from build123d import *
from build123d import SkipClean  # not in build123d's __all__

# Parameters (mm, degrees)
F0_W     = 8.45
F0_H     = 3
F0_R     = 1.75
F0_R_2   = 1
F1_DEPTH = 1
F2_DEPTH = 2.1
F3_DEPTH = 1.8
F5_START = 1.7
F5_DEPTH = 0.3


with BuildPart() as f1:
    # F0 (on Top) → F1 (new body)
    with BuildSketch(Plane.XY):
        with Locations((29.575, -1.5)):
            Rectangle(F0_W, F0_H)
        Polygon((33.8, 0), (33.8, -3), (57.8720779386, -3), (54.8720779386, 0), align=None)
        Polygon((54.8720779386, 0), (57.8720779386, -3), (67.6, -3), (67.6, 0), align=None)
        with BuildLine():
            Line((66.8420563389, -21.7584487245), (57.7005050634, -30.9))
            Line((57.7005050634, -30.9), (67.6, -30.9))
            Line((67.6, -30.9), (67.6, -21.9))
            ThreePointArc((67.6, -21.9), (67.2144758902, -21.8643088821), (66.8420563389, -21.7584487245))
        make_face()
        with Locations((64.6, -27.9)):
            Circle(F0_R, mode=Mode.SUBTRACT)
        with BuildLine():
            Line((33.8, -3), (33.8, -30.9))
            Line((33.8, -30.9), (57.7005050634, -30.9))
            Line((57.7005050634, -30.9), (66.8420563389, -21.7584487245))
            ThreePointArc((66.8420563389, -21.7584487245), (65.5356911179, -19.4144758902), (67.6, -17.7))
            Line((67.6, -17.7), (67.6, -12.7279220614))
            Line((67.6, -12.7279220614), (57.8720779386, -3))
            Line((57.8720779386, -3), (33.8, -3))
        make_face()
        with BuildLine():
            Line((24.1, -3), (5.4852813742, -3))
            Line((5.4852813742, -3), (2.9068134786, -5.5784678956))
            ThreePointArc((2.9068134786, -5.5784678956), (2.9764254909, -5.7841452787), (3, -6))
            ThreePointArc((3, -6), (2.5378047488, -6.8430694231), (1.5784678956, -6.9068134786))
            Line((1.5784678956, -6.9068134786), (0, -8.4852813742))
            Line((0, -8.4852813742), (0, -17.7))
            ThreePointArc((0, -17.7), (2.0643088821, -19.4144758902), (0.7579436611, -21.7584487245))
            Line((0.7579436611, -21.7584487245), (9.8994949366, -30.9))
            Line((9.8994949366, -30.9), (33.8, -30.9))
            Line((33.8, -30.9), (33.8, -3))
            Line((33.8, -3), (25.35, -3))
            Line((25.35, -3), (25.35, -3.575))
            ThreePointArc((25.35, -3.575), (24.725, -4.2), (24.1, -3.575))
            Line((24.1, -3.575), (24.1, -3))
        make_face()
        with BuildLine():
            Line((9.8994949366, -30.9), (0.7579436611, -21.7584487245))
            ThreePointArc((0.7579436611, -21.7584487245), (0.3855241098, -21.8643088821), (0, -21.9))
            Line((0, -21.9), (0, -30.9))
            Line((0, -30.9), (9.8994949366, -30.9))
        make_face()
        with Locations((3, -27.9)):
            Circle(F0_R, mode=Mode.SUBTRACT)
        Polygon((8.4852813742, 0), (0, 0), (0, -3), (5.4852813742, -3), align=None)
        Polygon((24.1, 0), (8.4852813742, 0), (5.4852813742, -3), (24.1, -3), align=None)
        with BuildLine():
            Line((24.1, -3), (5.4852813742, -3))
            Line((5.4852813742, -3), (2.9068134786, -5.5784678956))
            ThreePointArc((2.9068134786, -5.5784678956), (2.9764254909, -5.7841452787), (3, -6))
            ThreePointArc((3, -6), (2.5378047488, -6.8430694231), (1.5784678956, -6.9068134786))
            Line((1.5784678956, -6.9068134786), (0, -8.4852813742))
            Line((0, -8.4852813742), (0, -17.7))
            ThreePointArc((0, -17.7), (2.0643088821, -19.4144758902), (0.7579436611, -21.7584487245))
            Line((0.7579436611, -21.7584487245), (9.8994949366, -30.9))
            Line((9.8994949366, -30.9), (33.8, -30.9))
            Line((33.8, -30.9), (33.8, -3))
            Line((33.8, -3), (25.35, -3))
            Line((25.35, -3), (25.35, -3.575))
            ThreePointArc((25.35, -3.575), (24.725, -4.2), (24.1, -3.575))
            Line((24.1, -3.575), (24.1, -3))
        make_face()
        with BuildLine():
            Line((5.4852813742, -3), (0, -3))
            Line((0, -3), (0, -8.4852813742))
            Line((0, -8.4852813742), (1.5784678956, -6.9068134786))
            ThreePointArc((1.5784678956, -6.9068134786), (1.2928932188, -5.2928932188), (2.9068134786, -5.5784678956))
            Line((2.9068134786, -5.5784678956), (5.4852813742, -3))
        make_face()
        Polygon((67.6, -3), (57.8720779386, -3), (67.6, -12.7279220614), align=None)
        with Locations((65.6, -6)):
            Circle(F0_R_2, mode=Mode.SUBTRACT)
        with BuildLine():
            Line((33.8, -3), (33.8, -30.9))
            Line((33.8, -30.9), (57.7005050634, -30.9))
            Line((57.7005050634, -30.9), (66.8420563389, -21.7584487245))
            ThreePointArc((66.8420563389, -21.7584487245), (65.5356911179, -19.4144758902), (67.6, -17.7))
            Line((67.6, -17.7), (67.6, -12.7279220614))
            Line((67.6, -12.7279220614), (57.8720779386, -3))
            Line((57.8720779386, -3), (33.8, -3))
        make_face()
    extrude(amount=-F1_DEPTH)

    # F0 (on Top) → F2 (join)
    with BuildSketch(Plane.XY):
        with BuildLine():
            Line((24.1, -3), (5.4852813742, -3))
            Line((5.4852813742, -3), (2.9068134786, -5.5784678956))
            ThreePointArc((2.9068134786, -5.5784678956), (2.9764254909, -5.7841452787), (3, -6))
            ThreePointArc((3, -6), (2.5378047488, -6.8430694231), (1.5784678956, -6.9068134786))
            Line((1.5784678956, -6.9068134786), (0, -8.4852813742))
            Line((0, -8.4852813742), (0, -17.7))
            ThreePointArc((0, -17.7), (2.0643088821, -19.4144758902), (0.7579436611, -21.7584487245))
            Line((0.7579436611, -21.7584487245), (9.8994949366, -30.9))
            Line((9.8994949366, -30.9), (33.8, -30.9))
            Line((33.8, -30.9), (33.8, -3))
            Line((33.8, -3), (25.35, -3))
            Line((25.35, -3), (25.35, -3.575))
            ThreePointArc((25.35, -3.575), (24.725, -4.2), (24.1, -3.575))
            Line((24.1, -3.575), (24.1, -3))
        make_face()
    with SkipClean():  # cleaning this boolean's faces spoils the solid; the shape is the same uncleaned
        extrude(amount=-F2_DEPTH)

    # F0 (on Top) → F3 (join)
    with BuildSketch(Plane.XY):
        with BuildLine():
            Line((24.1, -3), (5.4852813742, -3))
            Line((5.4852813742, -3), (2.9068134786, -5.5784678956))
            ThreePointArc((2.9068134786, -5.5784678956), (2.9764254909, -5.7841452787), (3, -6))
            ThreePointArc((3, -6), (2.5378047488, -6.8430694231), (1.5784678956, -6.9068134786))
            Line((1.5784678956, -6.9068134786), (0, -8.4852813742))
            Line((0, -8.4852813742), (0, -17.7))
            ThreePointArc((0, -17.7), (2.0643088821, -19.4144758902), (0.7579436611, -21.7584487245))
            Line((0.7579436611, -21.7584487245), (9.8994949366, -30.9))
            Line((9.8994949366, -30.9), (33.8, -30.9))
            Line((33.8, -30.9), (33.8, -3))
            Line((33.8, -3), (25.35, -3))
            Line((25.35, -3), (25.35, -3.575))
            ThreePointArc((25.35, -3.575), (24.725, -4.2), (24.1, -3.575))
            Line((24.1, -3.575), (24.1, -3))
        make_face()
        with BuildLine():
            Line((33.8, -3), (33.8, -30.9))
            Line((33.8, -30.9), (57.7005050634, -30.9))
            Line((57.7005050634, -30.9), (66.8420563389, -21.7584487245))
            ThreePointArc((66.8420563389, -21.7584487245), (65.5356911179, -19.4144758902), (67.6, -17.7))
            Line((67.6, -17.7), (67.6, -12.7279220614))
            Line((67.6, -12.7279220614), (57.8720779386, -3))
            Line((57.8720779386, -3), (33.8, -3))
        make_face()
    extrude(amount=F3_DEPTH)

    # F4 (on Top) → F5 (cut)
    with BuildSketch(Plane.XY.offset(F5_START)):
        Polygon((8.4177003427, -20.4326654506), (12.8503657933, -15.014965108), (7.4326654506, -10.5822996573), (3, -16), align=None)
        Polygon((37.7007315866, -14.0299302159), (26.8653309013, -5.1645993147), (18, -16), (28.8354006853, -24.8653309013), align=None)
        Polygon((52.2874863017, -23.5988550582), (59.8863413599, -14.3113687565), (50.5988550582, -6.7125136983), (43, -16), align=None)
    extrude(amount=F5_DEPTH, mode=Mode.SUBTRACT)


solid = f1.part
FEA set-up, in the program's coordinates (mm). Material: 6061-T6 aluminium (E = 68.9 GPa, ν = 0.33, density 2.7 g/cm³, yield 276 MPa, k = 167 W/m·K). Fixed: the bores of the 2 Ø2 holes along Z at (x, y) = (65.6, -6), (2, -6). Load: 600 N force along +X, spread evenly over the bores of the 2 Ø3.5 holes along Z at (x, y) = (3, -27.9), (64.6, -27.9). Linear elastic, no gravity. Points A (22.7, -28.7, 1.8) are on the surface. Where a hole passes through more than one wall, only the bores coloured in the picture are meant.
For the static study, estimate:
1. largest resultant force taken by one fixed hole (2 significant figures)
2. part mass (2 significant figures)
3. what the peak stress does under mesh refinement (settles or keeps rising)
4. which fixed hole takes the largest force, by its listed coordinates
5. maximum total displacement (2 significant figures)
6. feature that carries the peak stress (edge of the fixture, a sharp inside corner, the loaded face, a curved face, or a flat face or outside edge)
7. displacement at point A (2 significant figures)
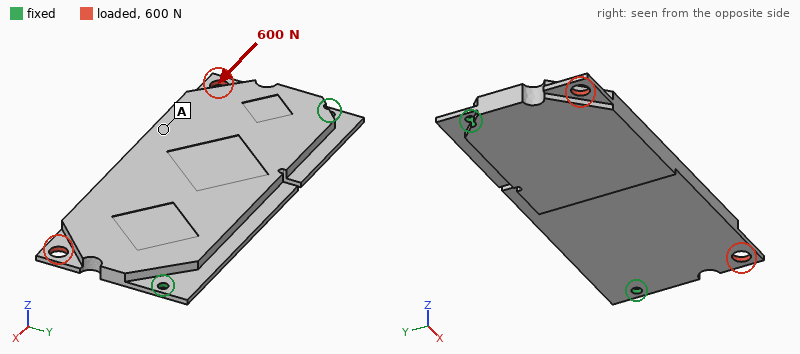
430 N
16 g
keeps rising
(2, -6)
55 µm
edge of the fixture
9.5 µm
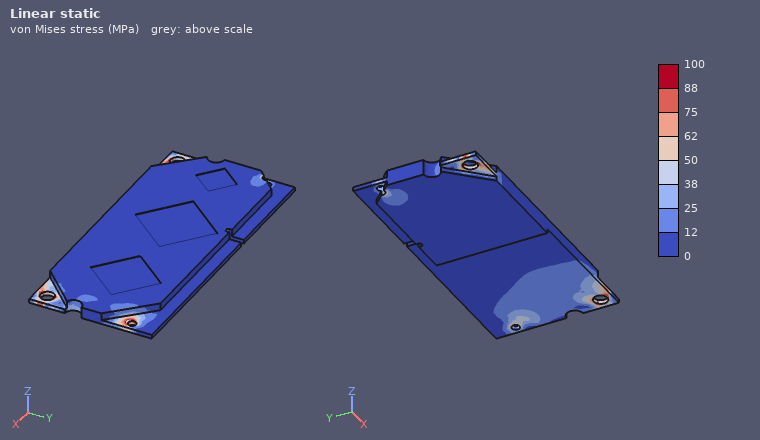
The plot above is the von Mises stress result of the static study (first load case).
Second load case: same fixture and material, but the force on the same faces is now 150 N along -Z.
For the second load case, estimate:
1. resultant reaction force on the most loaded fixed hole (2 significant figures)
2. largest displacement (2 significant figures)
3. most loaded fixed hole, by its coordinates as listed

86 N
0.47 mm
(2, -6)
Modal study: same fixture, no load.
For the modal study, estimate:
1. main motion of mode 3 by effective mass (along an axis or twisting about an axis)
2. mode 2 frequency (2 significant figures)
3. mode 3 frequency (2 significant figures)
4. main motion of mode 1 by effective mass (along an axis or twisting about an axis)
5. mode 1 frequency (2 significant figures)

twisting about Y
3700 Hz
4400 Hz
along Z
1500 Hz
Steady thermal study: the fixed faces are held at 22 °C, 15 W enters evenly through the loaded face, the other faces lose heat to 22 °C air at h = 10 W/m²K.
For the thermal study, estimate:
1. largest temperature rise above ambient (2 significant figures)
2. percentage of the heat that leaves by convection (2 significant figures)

59 K
5.3 %
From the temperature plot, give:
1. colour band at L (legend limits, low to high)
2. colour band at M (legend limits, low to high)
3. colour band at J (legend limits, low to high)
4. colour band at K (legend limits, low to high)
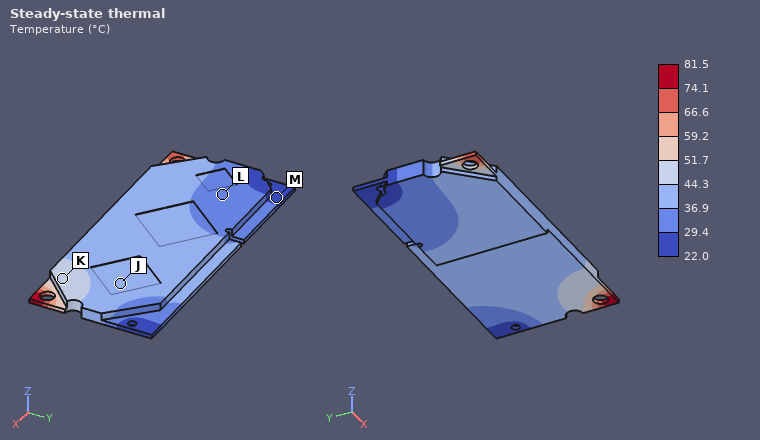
29.4 to 36.9 °C
22.0 to 29.4 °C
36.9 to 44.3 °C
44.3 to 51.7 °C
